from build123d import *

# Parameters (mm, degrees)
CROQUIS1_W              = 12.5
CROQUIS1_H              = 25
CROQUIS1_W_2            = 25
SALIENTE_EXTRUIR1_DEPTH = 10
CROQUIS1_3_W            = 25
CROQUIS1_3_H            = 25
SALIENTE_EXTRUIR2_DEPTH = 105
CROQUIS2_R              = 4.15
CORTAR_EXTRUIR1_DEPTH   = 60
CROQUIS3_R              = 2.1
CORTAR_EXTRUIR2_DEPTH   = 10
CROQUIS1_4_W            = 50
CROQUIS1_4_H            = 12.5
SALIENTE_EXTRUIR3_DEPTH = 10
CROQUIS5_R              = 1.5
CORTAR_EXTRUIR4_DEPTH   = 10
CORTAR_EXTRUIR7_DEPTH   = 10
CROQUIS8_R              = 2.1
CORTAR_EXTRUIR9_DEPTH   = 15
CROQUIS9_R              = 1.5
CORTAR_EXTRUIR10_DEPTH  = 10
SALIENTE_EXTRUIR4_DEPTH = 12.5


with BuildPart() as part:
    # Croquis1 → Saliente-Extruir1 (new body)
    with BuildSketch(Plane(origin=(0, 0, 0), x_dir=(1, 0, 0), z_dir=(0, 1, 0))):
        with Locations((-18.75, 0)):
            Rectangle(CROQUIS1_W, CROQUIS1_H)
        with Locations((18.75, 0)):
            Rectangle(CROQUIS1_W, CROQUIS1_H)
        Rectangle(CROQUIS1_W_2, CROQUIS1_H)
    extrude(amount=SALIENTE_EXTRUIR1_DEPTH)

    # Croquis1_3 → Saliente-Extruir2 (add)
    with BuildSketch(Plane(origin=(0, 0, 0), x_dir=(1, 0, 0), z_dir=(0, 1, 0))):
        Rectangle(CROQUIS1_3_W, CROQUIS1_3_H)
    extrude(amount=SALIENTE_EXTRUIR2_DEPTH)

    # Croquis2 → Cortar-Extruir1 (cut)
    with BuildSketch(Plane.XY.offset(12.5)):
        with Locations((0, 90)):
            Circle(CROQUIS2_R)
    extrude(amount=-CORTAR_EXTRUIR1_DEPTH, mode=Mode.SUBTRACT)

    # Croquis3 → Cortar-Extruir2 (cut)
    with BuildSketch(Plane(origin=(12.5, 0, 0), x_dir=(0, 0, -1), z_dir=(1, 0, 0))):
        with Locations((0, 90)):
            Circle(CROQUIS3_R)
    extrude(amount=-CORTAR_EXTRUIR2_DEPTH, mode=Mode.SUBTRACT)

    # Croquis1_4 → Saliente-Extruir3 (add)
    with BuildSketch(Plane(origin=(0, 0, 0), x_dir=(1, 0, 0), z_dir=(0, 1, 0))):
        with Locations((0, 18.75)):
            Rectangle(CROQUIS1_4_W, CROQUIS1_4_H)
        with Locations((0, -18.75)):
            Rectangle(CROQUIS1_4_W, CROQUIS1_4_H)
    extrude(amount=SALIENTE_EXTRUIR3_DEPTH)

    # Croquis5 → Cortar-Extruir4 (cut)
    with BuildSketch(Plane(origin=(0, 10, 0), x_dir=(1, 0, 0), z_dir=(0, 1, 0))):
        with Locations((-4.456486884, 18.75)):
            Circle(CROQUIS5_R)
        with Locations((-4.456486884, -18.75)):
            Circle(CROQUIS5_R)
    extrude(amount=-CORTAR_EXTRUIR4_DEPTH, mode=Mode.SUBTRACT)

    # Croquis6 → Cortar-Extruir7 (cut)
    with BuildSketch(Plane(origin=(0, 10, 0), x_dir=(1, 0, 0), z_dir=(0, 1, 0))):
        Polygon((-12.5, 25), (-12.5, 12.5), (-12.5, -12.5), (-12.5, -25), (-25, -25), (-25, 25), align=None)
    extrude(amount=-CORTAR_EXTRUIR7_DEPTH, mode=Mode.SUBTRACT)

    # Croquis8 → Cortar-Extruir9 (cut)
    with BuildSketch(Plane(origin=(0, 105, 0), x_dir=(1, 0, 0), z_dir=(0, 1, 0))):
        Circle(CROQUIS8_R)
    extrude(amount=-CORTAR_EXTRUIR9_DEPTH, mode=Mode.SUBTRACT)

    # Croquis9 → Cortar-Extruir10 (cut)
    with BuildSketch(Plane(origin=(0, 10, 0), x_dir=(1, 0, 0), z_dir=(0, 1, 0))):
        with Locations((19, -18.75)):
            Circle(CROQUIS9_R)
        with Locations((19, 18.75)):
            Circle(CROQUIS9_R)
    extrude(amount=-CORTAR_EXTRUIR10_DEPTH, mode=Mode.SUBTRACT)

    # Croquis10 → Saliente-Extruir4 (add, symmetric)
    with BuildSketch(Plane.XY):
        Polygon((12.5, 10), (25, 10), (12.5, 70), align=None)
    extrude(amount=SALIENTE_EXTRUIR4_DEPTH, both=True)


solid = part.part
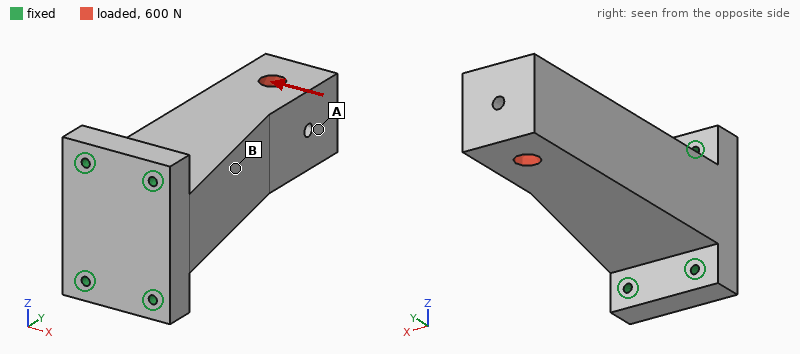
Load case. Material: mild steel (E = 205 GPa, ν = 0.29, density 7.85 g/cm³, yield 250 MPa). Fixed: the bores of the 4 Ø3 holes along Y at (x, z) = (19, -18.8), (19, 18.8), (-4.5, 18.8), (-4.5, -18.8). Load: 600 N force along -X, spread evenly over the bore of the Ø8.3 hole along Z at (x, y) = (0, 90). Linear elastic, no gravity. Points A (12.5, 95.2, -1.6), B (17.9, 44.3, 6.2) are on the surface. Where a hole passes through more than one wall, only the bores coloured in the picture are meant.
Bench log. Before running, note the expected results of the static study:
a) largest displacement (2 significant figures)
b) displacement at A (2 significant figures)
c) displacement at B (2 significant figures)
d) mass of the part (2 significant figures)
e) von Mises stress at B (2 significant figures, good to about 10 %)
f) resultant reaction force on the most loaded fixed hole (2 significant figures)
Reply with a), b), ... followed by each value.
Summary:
a) 22 µm
b) 19 µm
c) 6.4 µm
d) 670 g
e) 7.5 MPa
f) 970 N
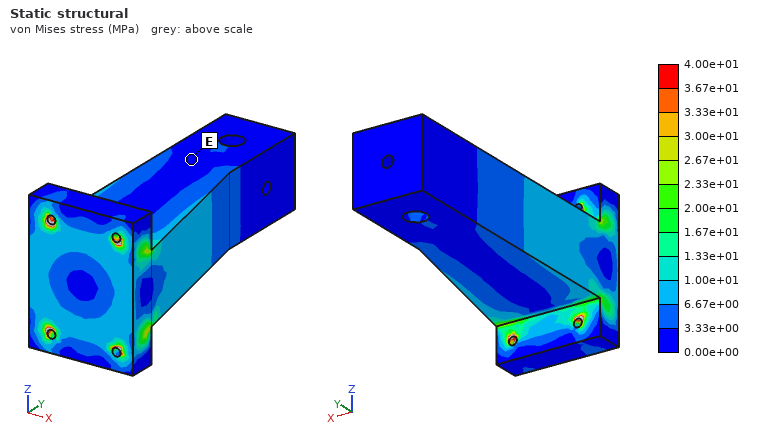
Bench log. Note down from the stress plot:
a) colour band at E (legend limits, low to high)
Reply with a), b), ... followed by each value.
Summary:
a) 0.00e+00 to 3.33e+00 MPa
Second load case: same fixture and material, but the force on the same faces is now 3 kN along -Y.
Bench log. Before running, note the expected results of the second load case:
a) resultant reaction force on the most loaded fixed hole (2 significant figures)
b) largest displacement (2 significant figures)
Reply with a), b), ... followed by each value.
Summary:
a) 1.2 kN
b) 8.0 µm
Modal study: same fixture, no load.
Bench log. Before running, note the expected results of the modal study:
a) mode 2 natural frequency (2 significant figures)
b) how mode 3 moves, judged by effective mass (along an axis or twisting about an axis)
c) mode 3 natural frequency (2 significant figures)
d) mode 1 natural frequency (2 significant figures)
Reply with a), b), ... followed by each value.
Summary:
a) 2100 Hz
b) twisting about Y
c) 8700 Hz
d) 2100 Hz
